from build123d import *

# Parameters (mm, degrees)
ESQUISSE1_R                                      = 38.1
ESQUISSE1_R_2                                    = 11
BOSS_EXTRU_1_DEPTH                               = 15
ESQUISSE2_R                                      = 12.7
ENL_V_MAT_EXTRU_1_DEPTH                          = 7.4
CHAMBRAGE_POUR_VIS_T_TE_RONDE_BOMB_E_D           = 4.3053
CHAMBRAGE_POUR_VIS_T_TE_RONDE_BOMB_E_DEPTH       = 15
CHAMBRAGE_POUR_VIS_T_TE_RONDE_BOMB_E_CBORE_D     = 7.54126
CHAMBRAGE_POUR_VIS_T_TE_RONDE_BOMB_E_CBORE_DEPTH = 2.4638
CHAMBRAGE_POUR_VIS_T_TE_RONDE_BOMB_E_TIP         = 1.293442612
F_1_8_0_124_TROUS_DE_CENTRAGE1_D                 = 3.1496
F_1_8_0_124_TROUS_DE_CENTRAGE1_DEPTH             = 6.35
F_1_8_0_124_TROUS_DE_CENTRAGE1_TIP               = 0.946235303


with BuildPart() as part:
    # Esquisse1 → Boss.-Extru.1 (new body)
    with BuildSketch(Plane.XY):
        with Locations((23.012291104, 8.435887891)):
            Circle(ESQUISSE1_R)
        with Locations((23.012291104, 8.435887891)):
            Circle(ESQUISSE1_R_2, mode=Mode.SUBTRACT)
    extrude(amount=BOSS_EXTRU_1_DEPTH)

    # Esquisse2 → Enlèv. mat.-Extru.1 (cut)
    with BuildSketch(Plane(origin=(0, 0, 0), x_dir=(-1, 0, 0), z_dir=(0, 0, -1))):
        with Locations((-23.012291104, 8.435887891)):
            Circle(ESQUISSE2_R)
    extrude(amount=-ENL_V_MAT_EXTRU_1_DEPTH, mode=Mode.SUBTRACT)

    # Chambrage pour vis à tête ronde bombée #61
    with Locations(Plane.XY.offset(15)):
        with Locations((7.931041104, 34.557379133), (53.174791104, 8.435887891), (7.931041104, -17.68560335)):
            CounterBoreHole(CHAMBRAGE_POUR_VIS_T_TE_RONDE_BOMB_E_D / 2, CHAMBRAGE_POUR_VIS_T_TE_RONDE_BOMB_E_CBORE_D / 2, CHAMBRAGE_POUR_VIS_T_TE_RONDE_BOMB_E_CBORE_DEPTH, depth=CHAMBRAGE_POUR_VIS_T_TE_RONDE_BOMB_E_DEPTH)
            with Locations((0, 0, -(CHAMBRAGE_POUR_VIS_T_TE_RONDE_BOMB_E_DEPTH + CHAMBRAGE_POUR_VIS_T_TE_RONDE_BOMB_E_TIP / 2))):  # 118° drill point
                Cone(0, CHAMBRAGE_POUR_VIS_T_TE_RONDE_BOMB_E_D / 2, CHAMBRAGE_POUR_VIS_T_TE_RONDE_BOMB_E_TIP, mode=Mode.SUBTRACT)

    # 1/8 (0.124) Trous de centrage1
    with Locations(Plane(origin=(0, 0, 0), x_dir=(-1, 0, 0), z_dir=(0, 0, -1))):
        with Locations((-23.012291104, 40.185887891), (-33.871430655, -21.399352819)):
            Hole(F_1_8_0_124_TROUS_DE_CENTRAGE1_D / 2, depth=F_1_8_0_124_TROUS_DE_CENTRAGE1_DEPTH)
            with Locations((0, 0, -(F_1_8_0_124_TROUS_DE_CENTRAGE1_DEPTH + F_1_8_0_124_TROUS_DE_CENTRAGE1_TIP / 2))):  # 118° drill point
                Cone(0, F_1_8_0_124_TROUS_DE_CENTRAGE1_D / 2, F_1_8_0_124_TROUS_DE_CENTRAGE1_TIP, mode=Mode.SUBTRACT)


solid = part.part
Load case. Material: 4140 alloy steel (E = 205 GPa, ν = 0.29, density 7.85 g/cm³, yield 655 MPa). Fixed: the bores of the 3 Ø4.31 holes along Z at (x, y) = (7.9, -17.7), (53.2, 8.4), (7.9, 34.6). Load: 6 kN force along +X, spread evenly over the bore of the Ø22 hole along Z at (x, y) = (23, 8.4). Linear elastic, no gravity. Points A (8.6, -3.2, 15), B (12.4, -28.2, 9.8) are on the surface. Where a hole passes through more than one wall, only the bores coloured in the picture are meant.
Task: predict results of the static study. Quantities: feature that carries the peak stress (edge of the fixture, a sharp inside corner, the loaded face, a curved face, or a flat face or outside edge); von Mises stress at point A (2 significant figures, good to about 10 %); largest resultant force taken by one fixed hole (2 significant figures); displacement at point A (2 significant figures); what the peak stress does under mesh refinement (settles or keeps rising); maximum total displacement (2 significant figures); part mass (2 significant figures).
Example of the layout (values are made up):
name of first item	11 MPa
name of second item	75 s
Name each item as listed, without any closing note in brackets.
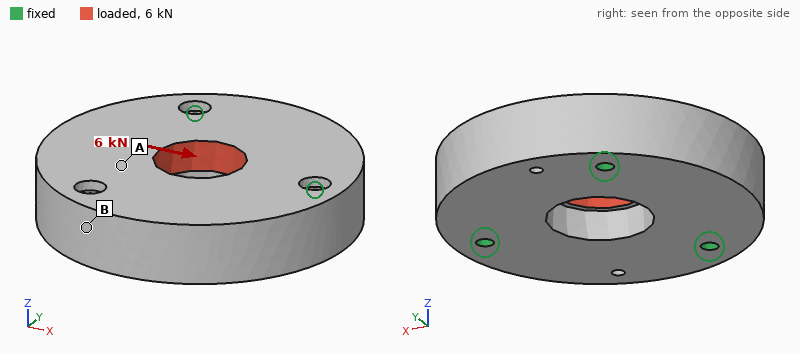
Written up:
feature that carries the peak stress	edge of the fixture
von Mises stress at point A	9.1 MPa
largest resultant force taken by one fixed hole	2.0 kN
displacement at point A	1.4 µm
what the peak stress does under mesh refinement	keeps rising
maximum total displacement	2.2 µm
part mass	480 g
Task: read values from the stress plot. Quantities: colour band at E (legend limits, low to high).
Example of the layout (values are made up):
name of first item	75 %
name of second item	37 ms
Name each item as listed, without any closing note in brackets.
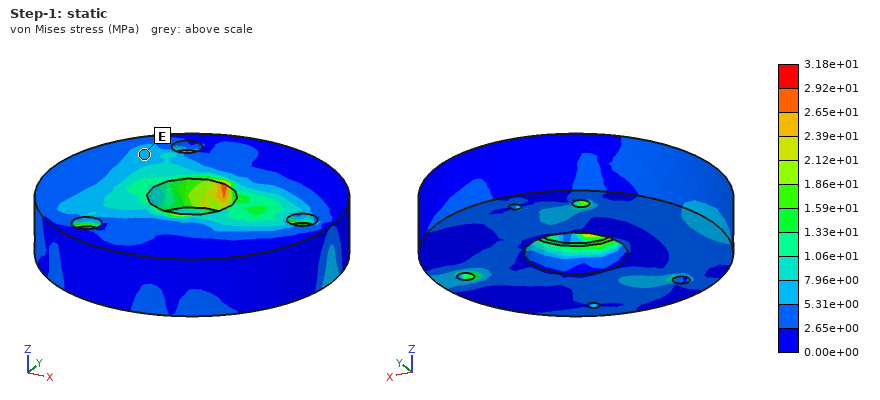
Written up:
colour band at E	5.31e+00 to 7.96e+00 MPa
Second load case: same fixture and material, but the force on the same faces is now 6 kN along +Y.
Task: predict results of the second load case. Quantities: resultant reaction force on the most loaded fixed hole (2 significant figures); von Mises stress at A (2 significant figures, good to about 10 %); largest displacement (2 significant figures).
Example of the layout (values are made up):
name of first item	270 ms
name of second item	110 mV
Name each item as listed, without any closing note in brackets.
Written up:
resultant reaction force on the most loaded fixed hole	2.1 kN
von Mises stress at A	8.7 MPa
largest displacement	2.0 µm
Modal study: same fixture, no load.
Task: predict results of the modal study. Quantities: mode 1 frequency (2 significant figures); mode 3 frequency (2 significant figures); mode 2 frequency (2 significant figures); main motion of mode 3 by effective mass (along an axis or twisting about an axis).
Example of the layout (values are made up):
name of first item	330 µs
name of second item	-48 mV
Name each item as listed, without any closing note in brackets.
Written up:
mode 1 frequency	11 kHz
mode 3 frequency	14 kHz
mode 2 frequency	11 kHz
main motion of mode 3 by effective mass	along Z
